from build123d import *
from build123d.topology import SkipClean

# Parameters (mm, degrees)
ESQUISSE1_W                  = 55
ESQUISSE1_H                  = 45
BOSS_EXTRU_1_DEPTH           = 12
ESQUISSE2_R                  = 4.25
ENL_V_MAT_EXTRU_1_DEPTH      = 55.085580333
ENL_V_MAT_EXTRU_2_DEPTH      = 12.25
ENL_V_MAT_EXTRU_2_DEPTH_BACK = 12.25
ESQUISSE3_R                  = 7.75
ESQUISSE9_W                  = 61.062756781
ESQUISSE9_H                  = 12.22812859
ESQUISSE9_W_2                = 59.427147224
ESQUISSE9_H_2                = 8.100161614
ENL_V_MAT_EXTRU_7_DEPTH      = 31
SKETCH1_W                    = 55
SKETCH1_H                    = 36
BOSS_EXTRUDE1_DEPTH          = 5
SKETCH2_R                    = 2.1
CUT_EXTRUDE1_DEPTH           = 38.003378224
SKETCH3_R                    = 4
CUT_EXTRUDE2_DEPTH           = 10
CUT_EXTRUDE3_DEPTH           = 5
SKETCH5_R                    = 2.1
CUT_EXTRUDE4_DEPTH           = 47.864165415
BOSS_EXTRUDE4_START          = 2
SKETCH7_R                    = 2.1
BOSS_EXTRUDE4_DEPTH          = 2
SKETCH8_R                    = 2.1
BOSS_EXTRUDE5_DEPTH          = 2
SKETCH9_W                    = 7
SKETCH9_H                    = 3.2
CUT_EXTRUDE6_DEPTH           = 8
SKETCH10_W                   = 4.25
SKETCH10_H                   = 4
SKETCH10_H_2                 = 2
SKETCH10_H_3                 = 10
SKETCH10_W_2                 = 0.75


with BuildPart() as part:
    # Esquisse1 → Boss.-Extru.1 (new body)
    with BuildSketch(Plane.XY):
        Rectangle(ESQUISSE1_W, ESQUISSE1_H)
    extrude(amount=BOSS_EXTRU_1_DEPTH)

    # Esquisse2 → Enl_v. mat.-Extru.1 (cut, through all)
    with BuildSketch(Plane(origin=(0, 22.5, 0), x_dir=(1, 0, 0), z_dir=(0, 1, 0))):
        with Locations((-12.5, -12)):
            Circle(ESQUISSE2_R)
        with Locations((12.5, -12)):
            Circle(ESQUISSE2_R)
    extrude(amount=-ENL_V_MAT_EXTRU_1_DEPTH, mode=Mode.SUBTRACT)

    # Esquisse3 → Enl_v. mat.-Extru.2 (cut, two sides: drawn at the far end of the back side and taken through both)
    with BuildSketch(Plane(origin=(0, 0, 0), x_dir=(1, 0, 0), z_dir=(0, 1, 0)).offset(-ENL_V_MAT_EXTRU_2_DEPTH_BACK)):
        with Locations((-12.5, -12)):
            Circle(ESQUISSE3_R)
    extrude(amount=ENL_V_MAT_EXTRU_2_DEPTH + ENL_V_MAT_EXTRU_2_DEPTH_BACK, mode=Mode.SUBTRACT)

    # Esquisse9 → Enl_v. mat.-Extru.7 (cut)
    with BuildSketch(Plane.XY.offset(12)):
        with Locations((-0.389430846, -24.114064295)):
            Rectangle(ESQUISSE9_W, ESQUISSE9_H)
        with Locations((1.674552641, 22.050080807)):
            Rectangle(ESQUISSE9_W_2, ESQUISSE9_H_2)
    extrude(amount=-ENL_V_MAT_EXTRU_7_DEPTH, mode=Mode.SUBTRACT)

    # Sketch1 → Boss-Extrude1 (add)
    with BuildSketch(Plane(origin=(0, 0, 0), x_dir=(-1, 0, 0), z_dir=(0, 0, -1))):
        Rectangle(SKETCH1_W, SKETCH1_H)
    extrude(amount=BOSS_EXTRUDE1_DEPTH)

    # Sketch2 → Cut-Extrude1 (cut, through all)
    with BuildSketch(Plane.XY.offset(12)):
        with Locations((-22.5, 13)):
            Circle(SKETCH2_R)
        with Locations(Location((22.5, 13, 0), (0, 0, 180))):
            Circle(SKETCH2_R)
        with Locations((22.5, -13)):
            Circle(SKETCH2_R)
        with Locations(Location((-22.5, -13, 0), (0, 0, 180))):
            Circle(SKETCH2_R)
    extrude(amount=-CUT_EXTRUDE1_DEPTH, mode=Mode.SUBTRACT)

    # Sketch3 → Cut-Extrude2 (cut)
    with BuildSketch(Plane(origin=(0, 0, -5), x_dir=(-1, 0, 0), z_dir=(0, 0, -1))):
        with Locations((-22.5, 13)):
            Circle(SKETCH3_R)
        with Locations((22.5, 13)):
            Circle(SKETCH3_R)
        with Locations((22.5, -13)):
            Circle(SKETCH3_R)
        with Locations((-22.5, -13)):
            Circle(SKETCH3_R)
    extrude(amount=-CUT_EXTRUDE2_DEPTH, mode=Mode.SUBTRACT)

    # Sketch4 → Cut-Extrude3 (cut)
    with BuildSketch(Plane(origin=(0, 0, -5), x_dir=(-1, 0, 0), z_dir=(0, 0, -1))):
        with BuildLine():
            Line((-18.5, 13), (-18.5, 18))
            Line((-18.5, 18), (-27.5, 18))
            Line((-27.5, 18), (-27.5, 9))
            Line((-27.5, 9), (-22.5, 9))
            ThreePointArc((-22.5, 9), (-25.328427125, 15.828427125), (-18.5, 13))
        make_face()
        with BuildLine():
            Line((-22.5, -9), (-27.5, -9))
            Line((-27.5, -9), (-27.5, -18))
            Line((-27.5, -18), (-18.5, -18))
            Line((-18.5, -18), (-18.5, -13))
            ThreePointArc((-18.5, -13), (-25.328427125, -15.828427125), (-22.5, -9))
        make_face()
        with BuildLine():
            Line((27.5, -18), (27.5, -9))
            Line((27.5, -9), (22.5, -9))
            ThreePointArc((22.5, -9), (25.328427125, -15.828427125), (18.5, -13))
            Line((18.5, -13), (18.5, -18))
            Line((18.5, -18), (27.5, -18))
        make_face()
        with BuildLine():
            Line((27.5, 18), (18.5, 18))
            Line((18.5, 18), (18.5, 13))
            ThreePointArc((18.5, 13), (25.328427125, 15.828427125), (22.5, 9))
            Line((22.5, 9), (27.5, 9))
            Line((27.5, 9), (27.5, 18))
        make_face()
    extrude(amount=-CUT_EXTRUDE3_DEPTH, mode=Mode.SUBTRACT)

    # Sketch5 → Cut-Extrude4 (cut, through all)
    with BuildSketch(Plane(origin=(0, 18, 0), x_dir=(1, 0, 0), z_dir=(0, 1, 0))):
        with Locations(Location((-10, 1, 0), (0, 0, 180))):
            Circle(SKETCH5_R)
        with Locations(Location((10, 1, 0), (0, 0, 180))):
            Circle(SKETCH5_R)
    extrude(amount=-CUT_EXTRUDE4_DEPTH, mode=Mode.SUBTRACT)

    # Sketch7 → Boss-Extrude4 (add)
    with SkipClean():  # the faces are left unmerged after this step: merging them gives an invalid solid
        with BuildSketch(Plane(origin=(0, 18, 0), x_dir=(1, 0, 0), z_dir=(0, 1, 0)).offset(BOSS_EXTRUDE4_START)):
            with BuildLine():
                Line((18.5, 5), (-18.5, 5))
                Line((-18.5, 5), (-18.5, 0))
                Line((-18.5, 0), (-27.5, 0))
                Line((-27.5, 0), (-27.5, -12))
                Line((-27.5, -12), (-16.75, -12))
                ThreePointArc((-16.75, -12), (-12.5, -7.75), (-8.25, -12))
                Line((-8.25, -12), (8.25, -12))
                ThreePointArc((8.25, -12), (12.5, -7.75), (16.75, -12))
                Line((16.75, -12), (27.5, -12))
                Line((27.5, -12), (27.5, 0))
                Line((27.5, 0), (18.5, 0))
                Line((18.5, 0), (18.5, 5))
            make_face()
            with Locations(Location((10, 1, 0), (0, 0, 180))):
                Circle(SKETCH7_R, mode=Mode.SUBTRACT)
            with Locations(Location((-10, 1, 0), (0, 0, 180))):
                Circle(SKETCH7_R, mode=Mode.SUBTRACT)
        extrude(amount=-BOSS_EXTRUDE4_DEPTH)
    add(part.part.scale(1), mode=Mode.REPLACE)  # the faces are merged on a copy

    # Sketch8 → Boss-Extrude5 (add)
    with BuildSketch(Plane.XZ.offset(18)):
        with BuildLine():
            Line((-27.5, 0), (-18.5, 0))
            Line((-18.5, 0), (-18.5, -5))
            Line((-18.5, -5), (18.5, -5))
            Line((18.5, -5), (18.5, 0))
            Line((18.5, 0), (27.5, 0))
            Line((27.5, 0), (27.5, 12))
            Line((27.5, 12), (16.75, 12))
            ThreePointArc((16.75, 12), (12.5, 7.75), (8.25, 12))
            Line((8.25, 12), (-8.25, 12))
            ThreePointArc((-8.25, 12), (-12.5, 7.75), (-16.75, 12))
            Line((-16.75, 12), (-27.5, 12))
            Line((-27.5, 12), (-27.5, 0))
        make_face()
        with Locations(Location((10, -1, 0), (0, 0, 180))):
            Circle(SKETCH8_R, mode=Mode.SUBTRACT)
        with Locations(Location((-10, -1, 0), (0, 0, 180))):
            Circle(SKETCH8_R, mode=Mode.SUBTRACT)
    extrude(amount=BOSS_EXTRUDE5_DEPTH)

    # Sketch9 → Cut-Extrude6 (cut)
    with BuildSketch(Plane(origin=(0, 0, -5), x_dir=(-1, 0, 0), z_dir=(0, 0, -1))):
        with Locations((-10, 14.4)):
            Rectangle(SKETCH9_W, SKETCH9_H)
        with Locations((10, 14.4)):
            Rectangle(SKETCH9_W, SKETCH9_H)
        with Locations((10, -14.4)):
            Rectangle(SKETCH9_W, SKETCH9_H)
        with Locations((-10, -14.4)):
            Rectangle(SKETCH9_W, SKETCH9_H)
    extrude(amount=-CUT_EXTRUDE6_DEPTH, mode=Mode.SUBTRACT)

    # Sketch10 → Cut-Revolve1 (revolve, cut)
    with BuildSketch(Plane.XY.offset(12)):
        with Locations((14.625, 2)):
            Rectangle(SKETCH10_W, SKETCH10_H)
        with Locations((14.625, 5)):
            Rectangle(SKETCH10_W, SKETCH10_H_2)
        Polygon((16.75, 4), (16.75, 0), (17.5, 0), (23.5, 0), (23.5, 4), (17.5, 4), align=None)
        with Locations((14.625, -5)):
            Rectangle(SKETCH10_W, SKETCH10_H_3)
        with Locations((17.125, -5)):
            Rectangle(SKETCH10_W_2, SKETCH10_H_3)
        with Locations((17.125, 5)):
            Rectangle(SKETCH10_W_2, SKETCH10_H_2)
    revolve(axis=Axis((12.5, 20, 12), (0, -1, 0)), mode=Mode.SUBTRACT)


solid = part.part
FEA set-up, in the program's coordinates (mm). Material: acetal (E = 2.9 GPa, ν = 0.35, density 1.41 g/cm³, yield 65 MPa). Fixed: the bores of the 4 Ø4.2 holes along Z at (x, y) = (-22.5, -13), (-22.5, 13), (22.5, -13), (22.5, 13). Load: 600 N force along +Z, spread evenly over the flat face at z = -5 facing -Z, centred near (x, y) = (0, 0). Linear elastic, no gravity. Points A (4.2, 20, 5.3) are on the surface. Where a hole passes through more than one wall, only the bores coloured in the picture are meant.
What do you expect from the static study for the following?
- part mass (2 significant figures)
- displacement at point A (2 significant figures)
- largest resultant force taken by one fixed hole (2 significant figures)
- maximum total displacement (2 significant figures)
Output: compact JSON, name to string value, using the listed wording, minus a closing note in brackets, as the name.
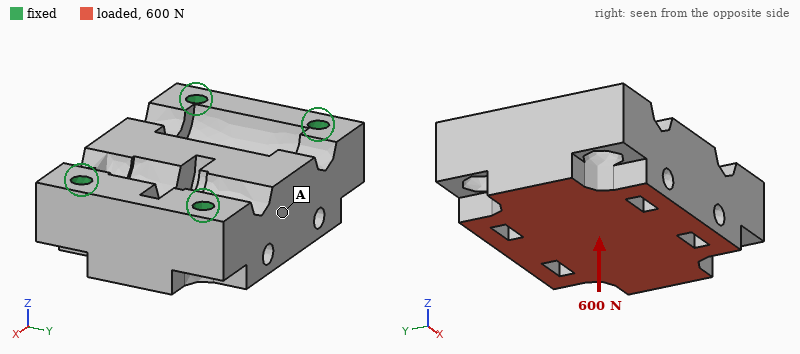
{"part mass": "39 g", "displacement at point A": "21 µm", "largest resultant force taken by one fixed hole": "180 N", "maximum total displacement": "22 µm"}
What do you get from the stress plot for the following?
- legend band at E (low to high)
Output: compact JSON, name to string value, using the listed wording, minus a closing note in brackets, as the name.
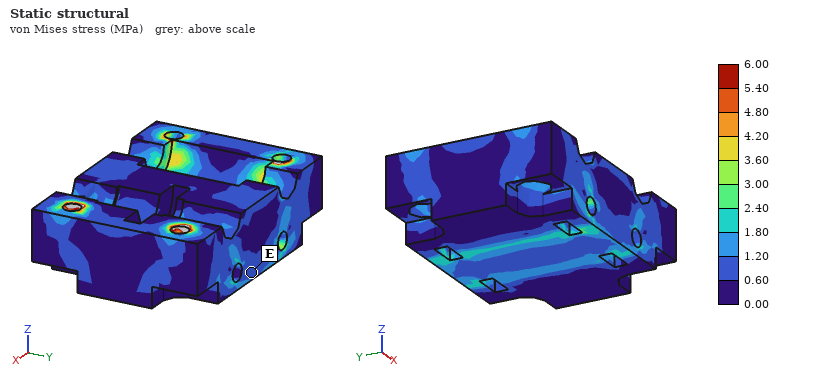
{"legend band at E": "0.60 to 1.20 MPa"}
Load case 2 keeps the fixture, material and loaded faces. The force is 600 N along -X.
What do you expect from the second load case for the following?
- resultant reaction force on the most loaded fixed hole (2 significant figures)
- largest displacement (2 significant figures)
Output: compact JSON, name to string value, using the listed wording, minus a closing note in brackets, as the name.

{"resultant reaction force on the most loaded fixed hole": "190 N", "largest displacement": "21 µm"}
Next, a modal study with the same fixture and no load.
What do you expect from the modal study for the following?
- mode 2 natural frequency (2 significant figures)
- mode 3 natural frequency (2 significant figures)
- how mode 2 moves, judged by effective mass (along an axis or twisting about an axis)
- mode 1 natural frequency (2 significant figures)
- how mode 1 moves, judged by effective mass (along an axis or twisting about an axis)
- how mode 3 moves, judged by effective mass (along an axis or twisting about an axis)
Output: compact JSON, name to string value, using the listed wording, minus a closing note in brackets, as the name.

{"mode 2 natural frequency": "5300 Hz", "mode 3 natural frequency": "5600 Hz", "how mode 2 moves, judged by effective mass": "along Y", "mode 1 natural frequency": "4700 Hz", "how mode 1 moves, judged by effective mass": "along Z", "how mode 3 moves, judged by effective mass": "along Y"}
